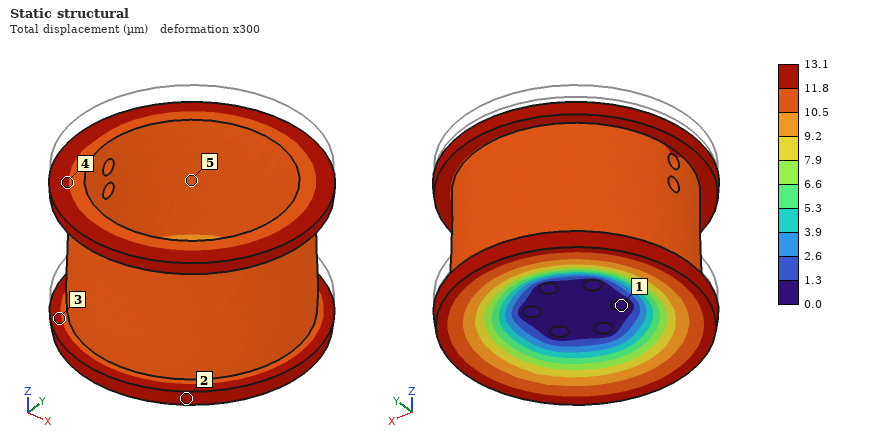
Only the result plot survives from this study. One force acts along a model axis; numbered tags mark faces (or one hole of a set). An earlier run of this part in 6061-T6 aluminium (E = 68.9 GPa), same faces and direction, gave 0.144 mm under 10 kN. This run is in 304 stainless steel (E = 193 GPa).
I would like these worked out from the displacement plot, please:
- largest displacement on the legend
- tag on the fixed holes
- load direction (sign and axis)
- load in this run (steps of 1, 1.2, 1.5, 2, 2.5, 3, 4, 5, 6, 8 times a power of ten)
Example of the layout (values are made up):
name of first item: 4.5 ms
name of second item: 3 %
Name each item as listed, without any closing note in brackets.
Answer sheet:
largest displacement on the legend: 13.1 µm
tag on the fixed holes: 1
load direction: -Z
load in this run: 2.5 kN
